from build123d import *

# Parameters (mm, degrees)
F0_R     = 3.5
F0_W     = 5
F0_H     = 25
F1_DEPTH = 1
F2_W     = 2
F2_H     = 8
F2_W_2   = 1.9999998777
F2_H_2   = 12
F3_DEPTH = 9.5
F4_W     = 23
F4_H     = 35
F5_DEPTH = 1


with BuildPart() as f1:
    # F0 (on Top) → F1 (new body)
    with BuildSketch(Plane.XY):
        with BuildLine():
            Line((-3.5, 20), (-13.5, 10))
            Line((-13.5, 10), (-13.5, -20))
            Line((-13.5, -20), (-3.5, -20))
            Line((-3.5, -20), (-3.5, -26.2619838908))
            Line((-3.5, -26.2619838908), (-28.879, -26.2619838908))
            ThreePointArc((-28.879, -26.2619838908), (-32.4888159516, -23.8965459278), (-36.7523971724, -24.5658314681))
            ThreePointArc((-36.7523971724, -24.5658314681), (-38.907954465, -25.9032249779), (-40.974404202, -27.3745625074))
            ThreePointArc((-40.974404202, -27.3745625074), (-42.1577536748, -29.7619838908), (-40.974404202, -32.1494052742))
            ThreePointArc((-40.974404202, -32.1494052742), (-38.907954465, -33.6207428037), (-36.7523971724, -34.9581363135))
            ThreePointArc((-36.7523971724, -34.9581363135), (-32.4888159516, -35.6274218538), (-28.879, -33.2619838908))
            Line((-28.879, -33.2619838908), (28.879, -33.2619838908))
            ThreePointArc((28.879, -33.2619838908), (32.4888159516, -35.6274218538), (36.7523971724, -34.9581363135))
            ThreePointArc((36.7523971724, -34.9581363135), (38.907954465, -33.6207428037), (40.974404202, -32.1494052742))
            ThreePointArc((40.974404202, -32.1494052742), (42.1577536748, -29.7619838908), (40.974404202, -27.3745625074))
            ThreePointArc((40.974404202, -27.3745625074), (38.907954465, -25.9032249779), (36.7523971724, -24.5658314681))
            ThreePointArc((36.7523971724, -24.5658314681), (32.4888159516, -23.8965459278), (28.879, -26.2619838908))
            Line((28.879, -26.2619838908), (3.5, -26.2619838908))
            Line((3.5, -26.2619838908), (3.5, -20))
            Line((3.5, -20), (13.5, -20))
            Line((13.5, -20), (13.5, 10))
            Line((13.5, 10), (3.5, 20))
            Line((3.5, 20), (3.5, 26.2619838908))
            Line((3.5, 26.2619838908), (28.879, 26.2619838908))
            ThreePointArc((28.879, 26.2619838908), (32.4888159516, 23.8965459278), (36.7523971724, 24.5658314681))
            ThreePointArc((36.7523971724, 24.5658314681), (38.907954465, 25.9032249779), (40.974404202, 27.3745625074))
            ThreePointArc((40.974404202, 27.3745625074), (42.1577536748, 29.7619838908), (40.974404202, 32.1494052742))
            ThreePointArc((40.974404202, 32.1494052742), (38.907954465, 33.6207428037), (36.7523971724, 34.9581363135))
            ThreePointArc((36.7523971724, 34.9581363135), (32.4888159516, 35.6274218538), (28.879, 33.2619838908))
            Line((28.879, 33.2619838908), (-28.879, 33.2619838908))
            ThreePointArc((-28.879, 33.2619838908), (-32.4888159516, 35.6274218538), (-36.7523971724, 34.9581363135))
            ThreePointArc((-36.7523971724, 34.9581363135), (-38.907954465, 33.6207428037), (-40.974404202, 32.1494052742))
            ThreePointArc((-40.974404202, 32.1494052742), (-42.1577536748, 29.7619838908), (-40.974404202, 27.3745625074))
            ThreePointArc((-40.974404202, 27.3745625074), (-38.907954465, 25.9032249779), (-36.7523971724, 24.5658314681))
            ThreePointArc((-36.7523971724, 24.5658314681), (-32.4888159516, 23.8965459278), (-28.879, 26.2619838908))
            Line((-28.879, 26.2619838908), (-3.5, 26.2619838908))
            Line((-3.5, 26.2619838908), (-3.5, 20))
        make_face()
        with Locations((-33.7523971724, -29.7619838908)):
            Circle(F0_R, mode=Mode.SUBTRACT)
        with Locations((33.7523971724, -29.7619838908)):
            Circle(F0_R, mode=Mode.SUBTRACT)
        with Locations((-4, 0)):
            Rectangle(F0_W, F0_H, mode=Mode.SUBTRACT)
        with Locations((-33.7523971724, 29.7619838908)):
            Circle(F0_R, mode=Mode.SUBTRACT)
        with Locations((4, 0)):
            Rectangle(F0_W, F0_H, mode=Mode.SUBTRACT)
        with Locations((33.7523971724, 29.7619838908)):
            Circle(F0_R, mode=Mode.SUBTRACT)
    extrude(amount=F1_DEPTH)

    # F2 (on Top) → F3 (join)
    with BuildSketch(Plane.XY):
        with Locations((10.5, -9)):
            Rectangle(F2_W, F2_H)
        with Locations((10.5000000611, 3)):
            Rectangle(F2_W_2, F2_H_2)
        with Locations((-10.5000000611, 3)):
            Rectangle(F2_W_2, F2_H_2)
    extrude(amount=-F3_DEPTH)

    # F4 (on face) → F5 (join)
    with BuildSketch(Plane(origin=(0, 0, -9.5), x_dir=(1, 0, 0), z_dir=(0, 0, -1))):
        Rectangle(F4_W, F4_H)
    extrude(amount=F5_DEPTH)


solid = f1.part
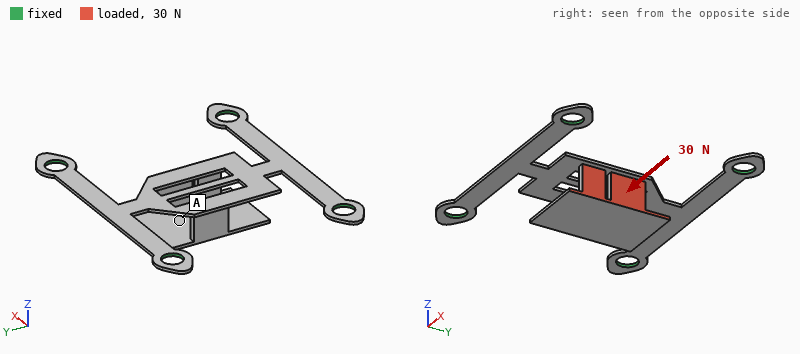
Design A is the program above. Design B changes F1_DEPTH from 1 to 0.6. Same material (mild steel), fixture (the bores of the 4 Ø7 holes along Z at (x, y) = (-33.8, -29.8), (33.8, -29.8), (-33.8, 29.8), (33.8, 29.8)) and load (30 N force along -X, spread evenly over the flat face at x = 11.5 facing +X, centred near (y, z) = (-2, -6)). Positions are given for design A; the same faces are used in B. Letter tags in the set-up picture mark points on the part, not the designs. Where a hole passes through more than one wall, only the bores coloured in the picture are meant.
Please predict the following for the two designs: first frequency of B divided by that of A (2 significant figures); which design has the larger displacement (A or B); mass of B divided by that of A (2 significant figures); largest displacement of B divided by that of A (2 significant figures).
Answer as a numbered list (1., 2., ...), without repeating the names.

1. 0.51
2. B
3. 0.77
4. 4.2
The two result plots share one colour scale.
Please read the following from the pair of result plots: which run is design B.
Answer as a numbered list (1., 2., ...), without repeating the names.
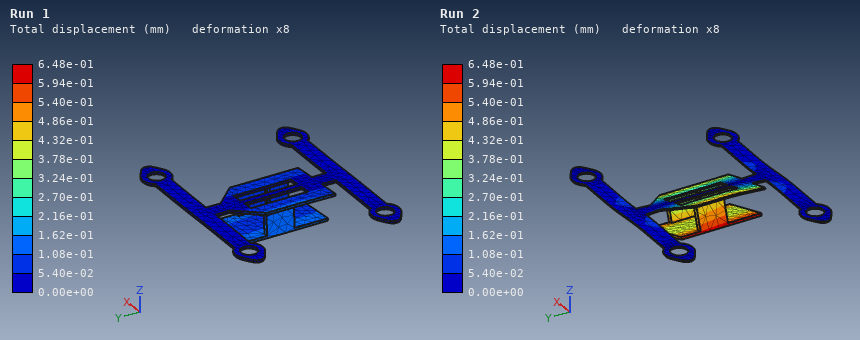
1. Run 2
